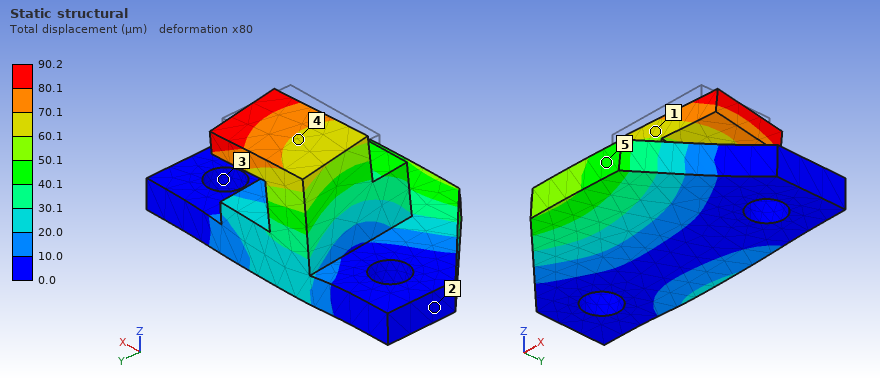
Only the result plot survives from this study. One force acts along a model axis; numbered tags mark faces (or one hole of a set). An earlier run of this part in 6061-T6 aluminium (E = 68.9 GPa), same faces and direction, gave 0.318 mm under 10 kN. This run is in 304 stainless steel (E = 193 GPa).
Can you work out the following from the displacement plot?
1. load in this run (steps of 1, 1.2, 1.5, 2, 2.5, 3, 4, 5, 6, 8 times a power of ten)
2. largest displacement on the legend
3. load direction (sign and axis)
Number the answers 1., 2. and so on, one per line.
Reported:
1. 8 kN
2. 90.2 µm
3. +Y
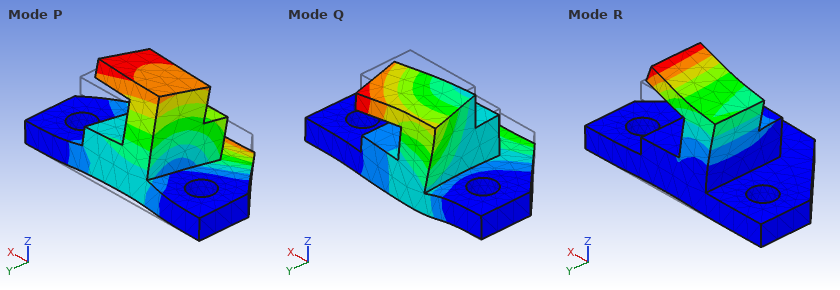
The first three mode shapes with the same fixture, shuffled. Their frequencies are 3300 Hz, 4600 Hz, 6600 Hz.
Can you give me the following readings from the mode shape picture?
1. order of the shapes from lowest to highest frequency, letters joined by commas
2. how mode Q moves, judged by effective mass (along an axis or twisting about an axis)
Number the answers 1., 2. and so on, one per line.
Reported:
1. P, R, Q
2. along Z
